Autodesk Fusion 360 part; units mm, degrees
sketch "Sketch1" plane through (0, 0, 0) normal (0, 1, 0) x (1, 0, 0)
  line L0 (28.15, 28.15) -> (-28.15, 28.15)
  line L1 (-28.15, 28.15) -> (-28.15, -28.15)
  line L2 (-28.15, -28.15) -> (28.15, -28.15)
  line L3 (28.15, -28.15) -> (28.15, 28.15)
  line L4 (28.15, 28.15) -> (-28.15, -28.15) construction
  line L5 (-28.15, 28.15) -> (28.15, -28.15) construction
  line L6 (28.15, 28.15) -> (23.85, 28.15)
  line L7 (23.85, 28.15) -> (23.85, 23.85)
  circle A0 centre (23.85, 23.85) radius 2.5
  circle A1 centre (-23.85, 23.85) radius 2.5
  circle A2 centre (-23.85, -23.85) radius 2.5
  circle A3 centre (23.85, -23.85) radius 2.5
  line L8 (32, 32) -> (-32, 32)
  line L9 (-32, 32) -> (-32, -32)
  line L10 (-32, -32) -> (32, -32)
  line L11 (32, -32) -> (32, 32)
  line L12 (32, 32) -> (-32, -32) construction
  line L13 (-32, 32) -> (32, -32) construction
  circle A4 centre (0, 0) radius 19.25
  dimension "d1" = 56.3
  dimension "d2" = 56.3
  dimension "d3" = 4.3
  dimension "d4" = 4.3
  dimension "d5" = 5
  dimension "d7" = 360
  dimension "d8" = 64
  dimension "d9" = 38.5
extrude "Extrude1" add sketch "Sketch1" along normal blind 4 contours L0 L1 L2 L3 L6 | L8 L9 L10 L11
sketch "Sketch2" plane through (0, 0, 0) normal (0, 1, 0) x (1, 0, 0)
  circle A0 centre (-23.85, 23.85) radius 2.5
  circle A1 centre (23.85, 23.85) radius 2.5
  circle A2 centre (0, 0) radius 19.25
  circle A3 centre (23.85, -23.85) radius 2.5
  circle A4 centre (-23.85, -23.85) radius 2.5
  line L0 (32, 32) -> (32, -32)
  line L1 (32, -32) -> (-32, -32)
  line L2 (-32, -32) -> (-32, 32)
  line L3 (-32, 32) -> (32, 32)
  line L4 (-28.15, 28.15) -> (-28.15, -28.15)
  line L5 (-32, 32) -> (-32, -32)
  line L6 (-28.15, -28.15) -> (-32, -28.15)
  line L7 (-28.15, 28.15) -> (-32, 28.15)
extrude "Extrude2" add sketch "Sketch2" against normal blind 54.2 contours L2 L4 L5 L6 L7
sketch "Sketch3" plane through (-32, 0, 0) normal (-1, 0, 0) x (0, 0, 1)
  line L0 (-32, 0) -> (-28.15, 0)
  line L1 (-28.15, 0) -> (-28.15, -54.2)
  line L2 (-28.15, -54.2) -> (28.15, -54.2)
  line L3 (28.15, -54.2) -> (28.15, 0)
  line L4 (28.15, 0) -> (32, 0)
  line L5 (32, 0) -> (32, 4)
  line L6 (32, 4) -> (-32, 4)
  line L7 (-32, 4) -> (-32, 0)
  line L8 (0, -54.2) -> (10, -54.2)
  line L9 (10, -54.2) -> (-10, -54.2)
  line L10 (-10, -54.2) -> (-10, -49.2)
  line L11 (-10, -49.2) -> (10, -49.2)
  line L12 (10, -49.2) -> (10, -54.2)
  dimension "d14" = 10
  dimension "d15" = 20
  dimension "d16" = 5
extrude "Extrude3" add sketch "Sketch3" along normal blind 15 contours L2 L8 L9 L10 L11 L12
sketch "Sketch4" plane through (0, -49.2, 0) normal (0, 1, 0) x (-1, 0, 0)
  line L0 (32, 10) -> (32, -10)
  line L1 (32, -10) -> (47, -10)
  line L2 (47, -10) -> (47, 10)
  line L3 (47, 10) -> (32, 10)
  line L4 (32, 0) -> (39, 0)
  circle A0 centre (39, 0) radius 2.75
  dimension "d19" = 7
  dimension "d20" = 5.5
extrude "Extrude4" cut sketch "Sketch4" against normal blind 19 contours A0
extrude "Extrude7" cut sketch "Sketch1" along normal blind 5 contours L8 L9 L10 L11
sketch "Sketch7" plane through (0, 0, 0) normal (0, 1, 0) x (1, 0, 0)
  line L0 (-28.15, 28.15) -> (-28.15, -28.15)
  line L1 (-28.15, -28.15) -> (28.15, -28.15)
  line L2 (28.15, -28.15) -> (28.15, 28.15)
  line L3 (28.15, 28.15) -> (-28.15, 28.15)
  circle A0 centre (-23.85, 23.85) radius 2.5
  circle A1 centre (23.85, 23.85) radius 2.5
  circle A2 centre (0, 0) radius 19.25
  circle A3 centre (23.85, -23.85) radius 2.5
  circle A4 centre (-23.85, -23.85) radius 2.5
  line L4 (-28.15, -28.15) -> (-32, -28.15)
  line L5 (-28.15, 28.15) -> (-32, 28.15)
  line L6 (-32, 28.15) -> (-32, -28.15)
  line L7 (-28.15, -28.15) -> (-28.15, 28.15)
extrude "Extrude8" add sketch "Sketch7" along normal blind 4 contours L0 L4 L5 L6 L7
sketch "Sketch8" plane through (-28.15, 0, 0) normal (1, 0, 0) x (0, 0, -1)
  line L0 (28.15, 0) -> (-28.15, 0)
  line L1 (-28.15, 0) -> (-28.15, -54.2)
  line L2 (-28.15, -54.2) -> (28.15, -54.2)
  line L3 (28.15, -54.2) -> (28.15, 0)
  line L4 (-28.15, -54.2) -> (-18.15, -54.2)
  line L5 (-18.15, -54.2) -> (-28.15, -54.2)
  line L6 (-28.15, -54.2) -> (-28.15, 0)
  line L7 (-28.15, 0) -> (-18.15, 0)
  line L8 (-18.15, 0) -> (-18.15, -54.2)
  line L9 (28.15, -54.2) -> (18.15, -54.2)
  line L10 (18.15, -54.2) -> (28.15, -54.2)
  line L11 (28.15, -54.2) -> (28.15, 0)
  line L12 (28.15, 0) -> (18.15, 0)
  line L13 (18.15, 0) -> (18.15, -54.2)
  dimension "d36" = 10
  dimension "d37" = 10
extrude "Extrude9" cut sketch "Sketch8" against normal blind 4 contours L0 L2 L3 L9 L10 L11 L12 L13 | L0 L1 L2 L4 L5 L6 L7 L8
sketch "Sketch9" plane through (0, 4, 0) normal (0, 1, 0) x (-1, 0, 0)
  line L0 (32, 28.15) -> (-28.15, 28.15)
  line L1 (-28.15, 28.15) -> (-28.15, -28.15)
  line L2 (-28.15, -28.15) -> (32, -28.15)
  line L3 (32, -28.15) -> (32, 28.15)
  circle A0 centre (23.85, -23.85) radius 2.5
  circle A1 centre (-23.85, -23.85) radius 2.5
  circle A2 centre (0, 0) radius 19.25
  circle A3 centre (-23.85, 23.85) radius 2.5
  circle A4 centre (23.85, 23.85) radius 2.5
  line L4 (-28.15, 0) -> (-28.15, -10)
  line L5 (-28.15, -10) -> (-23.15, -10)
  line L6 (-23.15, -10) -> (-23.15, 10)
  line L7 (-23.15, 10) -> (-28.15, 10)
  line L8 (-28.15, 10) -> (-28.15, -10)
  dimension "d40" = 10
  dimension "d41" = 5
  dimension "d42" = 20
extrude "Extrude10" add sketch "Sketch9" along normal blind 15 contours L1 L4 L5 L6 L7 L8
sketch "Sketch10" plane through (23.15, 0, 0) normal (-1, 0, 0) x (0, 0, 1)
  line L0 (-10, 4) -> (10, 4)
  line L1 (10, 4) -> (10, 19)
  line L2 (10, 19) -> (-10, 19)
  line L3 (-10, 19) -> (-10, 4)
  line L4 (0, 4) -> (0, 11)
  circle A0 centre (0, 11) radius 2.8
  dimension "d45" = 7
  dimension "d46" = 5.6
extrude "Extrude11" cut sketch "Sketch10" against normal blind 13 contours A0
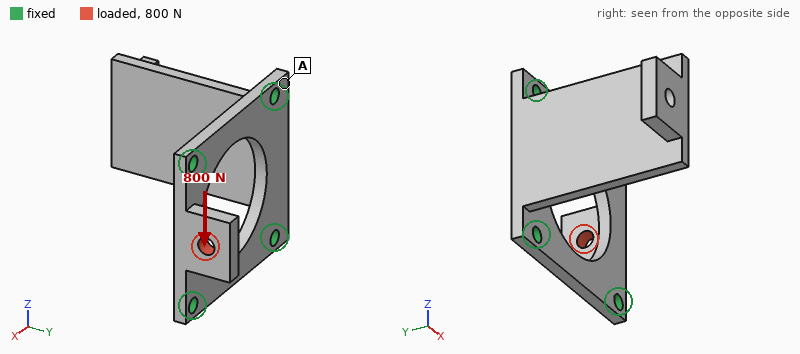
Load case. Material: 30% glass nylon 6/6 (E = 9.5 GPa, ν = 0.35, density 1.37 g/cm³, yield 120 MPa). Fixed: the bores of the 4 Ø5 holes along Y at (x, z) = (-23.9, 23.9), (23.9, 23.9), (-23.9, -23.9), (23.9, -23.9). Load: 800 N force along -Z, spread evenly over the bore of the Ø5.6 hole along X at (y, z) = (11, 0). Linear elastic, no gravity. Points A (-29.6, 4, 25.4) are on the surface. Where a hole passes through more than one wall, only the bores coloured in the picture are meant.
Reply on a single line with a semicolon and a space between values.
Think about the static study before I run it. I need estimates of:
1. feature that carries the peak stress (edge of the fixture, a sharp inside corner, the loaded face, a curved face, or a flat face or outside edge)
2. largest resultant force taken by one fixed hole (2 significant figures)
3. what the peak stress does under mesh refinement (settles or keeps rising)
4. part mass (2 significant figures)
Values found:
edge of the fixture; 450 N; keeps rising; 26 g
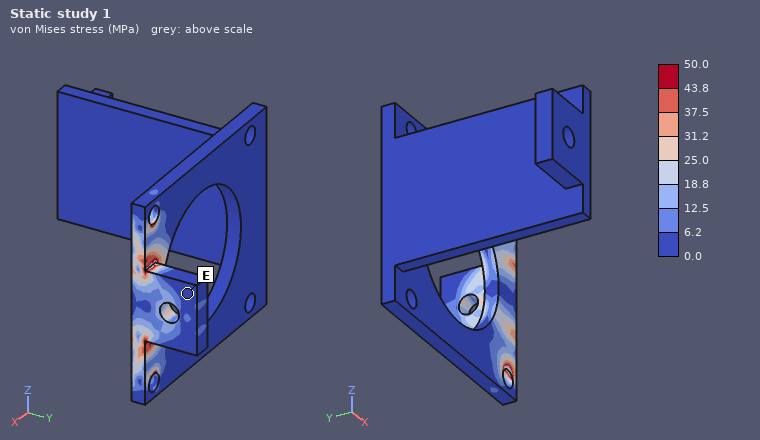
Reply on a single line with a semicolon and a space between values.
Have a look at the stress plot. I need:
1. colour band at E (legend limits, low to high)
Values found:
0.0 to 6.2 MPa
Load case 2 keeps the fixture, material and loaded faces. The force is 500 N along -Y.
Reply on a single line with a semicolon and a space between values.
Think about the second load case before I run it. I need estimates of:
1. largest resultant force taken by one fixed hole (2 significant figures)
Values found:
280 N
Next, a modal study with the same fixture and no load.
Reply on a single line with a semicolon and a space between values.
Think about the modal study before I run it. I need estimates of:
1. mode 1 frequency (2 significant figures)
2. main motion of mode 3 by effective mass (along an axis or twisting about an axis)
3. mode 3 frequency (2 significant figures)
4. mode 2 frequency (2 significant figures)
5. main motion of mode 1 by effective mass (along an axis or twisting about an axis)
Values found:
340 Hz; along Z; 1900 Hz; 1400 Hz; along X
